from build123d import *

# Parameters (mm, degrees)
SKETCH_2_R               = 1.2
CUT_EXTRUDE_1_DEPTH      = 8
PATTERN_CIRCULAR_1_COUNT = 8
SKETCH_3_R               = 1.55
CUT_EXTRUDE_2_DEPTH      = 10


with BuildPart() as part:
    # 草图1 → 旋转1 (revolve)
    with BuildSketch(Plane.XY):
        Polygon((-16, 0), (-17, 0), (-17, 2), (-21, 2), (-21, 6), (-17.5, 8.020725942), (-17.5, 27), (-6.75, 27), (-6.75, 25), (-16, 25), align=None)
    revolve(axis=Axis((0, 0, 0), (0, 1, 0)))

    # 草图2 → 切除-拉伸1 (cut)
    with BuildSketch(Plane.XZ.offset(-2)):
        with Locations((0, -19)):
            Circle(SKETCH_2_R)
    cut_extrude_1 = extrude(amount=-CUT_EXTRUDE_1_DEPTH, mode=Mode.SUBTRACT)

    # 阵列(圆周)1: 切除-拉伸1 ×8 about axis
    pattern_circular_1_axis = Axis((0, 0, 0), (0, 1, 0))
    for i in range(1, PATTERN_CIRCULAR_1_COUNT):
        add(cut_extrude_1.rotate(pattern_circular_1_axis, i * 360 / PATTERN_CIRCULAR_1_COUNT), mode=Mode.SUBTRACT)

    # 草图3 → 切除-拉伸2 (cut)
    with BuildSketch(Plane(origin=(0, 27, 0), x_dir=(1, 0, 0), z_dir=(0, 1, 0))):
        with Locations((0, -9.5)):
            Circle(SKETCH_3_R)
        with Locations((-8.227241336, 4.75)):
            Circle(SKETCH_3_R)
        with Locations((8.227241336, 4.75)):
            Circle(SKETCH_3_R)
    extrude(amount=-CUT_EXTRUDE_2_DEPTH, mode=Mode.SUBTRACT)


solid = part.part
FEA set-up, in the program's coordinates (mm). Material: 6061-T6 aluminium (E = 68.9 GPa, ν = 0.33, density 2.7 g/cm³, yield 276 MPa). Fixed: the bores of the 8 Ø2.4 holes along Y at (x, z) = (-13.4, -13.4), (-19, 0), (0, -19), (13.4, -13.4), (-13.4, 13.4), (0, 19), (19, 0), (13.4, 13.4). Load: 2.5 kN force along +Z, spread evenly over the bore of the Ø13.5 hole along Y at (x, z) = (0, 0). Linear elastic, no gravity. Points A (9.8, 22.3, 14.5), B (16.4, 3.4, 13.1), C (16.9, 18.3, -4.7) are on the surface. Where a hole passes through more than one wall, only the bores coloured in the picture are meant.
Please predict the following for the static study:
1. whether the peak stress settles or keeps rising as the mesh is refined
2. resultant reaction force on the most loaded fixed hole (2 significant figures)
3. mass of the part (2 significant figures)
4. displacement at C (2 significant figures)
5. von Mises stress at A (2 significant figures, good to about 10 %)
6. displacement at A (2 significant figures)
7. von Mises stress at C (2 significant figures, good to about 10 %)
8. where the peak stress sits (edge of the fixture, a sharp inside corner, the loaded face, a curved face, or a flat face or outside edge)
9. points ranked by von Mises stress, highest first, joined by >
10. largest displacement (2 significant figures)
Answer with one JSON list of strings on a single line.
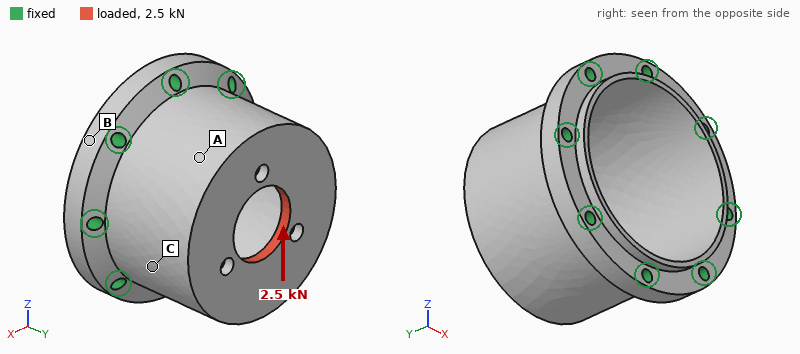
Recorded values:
["keeps rising", "730 N", "20 g", "16 µm", "35 MPa", "27 µm", "50 MPa", "edge of the fixture", "C > A > B", "47 µm"]
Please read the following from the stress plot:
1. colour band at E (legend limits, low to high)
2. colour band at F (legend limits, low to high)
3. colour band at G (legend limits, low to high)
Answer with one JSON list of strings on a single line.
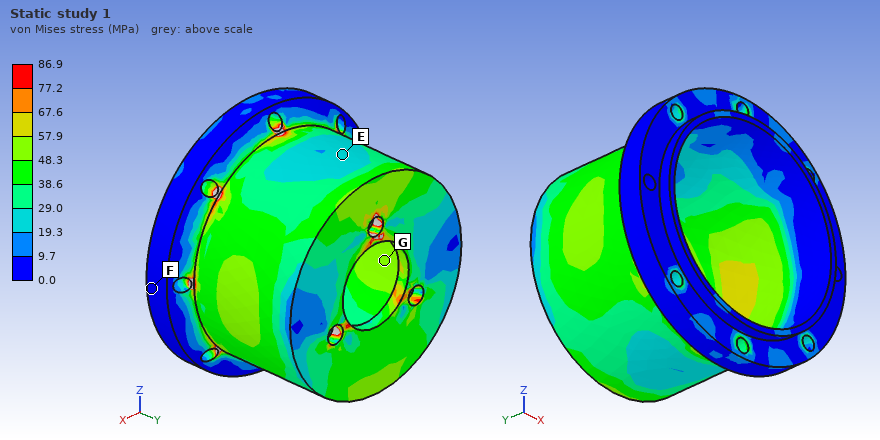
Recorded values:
["19.3 to 29.0 MPa", "0.0 to 9.7 MPa", "48.3 to 57.9 MPa"]
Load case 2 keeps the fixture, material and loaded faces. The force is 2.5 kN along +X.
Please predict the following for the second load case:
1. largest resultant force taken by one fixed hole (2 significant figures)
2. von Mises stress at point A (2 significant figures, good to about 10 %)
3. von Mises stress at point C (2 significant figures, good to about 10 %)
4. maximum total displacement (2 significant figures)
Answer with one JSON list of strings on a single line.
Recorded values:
["730 N", "39 MPa", "25 MPa", "45 µm"]
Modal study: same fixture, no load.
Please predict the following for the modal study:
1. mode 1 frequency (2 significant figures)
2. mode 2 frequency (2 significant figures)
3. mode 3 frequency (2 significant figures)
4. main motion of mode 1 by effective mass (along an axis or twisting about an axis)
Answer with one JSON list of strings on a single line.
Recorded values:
["16 kHz", "17 kHz", "17 kHz", "along Y"]
